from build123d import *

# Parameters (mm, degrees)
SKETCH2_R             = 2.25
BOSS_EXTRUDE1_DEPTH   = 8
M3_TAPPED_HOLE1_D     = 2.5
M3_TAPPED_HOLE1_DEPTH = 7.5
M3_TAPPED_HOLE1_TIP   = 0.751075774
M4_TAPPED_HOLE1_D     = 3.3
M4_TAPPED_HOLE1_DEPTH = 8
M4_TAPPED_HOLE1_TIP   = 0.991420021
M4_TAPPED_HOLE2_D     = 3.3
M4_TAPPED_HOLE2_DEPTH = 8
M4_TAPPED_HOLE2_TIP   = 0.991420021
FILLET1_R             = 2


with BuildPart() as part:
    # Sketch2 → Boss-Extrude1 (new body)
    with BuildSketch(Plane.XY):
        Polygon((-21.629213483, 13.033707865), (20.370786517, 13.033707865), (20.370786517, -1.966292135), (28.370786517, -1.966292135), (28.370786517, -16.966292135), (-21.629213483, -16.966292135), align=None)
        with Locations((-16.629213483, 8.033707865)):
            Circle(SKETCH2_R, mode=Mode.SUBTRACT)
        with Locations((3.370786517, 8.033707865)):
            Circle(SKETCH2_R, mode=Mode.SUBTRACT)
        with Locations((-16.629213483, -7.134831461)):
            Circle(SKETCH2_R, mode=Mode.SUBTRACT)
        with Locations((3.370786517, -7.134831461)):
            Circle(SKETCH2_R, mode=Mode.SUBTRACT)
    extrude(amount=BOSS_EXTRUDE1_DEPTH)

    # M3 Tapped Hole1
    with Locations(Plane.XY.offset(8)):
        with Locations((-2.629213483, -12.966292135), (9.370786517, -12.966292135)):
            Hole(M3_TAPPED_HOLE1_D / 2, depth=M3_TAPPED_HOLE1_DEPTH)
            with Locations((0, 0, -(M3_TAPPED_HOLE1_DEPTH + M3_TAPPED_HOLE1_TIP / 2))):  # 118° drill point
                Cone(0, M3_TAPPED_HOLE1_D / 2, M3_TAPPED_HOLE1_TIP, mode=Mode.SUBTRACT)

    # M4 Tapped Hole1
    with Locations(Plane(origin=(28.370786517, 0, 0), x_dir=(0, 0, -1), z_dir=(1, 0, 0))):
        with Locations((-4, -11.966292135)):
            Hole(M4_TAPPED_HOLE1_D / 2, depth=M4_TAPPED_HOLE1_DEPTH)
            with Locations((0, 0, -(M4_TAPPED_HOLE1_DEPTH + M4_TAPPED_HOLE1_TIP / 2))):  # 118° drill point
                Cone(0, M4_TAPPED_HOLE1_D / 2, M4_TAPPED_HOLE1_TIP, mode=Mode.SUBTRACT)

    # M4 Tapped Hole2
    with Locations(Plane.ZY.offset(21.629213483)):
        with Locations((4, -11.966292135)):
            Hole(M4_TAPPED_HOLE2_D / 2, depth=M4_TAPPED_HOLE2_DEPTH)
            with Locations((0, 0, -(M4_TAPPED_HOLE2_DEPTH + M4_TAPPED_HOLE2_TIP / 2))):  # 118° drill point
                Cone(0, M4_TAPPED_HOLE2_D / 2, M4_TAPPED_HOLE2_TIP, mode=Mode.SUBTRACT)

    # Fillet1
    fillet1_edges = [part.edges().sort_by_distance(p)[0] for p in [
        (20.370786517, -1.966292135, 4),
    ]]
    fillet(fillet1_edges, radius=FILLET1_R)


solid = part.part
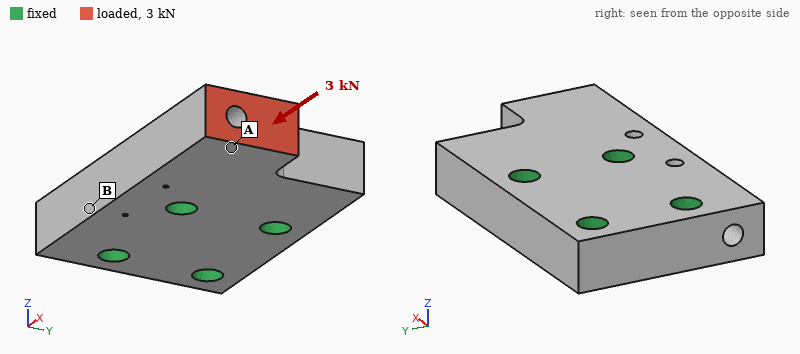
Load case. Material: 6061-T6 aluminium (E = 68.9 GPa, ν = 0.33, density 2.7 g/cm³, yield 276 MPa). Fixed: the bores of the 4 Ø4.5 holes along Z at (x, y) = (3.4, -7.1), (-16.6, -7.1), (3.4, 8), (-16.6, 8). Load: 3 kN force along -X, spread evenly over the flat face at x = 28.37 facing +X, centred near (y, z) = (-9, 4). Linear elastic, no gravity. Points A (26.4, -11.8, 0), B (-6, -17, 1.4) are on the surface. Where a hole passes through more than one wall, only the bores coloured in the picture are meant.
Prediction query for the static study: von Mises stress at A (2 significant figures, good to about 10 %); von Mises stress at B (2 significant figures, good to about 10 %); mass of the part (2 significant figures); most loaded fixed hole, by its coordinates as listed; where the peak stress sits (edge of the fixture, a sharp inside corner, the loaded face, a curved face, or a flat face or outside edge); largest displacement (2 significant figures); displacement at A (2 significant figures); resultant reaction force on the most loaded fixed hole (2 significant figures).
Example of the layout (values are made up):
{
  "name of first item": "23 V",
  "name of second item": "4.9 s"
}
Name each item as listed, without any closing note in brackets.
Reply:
{
  "von Mises stress at A": "27 MPa",
  "von Mises stress at B": "9.0 MPa",
  "mass of the part": "28 g",
  "most loaded fixed hole, by its coordinates as listed": "(3.4, -7.1)",
  "where the peak stress sits": "a curved face",
  "largest displacement": "16 µm",
  "displacement at A": "13 µm",
  "resultant reaction force on the most loaded fixed hole": "2.6 kN"
}
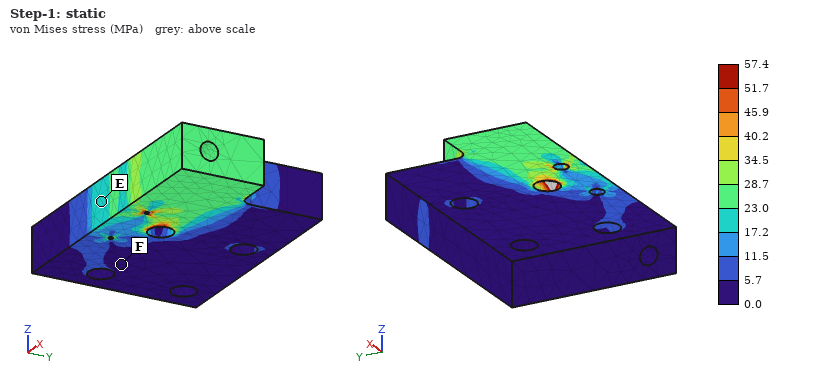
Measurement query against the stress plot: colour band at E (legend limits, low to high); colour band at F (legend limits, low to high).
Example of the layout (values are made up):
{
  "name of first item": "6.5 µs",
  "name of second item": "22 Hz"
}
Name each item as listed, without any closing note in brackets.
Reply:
{
  "colour band at E": "17.2 to 23.0 MPa",
  "colour band at F": "0.0 to 5.7 MPa"
}
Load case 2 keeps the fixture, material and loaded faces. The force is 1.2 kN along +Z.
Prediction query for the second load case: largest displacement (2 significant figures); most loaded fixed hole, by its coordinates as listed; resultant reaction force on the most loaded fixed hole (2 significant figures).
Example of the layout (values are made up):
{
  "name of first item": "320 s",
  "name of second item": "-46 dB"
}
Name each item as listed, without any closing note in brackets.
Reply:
{
  "largest displacement": "0.12 mm",
  "most loaded fixed hole, by its coordinates as listed": "(3.4, -7.1)",
  "resultant reaction force on the most loaded fixed hole": "1.3 kN"
}
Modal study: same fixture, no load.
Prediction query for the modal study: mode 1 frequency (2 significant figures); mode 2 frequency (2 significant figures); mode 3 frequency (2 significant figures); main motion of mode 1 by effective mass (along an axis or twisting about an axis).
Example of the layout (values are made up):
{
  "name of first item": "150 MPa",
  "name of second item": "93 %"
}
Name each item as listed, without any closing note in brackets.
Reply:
{
  "mode 1 frequency": "12 kHz",
  "mode 2 frequency": "24 kHz",
  "mode 3 frequency": "25 kHz",
  "main motion of mode 1 by effective mass": "along Z"
}
